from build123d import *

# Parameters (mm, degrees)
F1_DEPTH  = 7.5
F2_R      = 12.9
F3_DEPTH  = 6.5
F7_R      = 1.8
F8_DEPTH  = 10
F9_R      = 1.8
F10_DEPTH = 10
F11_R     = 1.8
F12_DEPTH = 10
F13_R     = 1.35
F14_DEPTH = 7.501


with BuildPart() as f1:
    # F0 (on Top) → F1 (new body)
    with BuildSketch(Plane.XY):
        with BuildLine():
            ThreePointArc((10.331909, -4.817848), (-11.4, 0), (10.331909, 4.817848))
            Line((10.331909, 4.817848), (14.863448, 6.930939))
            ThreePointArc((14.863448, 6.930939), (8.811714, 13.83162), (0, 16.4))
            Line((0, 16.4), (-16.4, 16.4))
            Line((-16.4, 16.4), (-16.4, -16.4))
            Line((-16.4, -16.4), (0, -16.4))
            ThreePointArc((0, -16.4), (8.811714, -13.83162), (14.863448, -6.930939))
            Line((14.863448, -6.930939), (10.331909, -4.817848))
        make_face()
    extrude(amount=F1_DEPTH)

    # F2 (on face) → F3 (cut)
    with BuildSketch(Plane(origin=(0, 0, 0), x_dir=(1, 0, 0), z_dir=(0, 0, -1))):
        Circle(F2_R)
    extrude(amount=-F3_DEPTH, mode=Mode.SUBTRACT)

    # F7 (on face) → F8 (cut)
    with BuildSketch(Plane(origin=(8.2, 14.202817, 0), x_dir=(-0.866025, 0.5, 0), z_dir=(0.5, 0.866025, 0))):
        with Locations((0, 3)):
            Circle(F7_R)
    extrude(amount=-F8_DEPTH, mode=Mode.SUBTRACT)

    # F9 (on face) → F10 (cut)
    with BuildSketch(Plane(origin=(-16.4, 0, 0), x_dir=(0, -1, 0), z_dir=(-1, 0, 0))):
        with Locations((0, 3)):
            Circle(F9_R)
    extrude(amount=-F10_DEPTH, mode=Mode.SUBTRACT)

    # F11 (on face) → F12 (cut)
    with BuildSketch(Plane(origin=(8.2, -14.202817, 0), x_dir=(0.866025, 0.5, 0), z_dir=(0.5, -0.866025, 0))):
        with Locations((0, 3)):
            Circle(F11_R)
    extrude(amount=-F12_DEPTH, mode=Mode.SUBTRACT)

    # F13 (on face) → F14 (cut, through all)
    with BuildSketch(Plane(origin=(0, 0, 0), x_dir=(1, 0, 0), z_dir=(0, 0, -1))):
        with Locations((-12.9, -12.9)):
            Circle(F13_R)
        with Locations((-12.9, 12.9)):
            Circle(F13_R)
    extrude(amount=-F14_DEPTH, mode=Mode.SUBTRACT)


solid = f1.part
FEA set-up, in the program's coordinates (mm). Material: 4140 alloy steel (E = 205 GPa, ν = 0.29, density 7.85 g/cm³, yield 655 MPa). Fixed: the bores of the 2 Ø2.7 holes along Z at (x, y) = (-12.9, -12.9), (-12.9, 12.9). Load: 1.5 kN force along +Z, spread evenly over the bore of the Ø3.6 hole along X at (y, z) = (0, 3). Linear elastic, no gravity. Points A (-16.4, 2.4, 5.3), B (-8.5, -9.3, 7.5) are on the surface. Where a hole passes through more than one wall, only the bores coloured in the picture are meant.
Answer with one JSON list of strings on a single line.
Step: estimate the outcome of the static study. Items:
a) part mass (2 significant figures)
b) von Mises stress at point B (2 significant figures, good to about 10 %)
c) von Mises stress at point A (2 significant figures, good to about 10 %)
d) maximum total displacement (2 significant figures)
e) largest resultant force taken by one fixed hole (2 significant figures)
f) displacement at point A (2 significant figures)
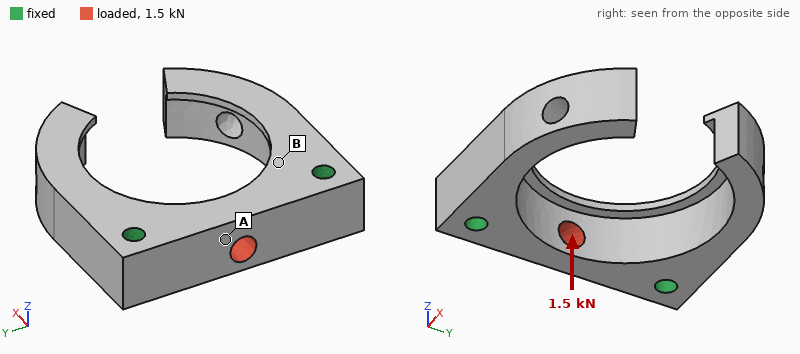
["22 g", "23 MPa", "57 MPa", "8.1 µm", "760 N", "6.2 µm"]
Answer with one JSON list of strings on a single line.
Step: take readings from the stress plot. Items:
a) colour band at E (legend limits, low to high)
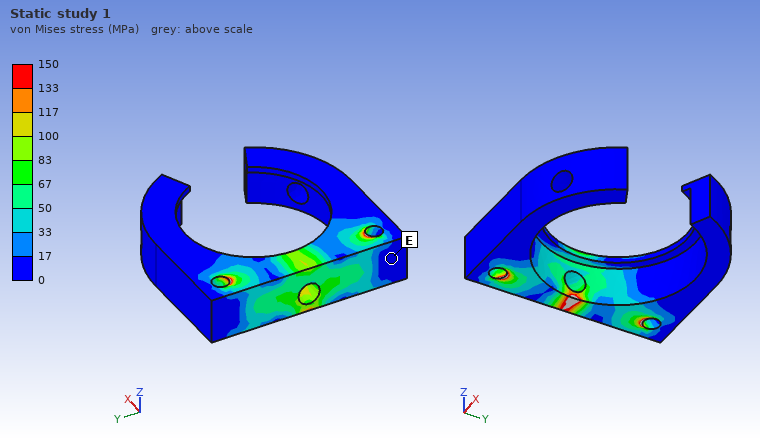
["0 to 17 MPa"]
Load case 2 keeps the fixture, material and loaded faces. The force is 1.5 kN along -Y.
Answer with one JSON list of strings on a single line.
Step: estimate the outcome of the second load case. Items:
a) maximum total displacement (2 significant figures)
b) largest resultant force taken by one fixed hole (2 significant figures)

["1.7 µm", "760 N"]
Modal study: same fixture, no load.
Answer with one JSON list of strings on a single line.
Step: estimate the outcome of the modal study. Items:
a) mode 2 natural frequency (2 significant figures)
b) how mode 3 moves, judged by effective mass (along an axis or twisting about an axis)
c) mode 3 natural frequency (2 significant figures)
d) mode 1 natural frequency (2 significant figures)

["6000 Hz", "along Z", "8000 Hz", "5900 Hz"]
